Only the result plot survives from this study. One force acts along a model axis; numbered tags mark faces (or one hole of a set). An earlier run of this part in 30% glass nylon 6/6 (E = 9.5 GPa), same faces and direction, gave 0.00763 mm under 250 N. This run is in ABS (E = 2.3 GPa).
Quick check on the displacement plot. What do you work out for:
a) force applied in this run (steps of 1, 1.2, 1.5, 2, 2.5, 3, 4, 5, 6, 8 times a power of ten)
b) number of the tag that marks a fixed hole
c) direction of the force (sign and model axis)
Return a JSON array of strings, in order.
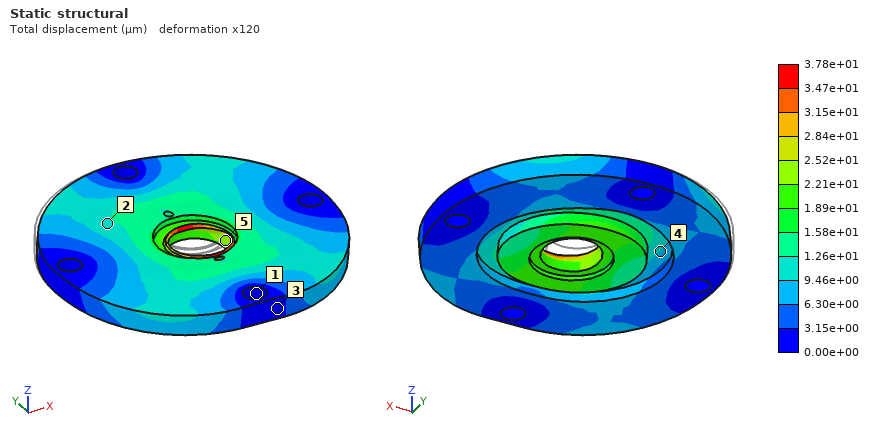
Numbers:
["300 N", "1", "-Y"]
